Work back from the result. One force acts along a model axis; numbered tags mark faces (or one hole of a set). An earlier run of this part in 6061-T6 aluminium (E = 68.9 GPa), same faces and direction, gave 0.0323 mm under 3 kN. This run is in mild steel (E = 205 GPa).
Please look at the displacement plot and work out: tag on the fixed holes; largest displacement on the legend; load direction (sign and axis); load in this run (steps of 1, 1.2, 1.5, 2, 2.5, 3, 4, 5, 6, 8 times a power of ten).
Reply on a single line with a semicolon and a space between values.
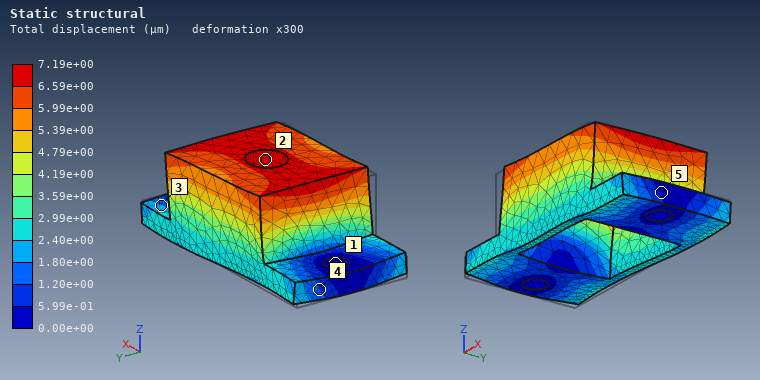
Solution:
1; 7.19e+00 µm; +X; 2 kN
